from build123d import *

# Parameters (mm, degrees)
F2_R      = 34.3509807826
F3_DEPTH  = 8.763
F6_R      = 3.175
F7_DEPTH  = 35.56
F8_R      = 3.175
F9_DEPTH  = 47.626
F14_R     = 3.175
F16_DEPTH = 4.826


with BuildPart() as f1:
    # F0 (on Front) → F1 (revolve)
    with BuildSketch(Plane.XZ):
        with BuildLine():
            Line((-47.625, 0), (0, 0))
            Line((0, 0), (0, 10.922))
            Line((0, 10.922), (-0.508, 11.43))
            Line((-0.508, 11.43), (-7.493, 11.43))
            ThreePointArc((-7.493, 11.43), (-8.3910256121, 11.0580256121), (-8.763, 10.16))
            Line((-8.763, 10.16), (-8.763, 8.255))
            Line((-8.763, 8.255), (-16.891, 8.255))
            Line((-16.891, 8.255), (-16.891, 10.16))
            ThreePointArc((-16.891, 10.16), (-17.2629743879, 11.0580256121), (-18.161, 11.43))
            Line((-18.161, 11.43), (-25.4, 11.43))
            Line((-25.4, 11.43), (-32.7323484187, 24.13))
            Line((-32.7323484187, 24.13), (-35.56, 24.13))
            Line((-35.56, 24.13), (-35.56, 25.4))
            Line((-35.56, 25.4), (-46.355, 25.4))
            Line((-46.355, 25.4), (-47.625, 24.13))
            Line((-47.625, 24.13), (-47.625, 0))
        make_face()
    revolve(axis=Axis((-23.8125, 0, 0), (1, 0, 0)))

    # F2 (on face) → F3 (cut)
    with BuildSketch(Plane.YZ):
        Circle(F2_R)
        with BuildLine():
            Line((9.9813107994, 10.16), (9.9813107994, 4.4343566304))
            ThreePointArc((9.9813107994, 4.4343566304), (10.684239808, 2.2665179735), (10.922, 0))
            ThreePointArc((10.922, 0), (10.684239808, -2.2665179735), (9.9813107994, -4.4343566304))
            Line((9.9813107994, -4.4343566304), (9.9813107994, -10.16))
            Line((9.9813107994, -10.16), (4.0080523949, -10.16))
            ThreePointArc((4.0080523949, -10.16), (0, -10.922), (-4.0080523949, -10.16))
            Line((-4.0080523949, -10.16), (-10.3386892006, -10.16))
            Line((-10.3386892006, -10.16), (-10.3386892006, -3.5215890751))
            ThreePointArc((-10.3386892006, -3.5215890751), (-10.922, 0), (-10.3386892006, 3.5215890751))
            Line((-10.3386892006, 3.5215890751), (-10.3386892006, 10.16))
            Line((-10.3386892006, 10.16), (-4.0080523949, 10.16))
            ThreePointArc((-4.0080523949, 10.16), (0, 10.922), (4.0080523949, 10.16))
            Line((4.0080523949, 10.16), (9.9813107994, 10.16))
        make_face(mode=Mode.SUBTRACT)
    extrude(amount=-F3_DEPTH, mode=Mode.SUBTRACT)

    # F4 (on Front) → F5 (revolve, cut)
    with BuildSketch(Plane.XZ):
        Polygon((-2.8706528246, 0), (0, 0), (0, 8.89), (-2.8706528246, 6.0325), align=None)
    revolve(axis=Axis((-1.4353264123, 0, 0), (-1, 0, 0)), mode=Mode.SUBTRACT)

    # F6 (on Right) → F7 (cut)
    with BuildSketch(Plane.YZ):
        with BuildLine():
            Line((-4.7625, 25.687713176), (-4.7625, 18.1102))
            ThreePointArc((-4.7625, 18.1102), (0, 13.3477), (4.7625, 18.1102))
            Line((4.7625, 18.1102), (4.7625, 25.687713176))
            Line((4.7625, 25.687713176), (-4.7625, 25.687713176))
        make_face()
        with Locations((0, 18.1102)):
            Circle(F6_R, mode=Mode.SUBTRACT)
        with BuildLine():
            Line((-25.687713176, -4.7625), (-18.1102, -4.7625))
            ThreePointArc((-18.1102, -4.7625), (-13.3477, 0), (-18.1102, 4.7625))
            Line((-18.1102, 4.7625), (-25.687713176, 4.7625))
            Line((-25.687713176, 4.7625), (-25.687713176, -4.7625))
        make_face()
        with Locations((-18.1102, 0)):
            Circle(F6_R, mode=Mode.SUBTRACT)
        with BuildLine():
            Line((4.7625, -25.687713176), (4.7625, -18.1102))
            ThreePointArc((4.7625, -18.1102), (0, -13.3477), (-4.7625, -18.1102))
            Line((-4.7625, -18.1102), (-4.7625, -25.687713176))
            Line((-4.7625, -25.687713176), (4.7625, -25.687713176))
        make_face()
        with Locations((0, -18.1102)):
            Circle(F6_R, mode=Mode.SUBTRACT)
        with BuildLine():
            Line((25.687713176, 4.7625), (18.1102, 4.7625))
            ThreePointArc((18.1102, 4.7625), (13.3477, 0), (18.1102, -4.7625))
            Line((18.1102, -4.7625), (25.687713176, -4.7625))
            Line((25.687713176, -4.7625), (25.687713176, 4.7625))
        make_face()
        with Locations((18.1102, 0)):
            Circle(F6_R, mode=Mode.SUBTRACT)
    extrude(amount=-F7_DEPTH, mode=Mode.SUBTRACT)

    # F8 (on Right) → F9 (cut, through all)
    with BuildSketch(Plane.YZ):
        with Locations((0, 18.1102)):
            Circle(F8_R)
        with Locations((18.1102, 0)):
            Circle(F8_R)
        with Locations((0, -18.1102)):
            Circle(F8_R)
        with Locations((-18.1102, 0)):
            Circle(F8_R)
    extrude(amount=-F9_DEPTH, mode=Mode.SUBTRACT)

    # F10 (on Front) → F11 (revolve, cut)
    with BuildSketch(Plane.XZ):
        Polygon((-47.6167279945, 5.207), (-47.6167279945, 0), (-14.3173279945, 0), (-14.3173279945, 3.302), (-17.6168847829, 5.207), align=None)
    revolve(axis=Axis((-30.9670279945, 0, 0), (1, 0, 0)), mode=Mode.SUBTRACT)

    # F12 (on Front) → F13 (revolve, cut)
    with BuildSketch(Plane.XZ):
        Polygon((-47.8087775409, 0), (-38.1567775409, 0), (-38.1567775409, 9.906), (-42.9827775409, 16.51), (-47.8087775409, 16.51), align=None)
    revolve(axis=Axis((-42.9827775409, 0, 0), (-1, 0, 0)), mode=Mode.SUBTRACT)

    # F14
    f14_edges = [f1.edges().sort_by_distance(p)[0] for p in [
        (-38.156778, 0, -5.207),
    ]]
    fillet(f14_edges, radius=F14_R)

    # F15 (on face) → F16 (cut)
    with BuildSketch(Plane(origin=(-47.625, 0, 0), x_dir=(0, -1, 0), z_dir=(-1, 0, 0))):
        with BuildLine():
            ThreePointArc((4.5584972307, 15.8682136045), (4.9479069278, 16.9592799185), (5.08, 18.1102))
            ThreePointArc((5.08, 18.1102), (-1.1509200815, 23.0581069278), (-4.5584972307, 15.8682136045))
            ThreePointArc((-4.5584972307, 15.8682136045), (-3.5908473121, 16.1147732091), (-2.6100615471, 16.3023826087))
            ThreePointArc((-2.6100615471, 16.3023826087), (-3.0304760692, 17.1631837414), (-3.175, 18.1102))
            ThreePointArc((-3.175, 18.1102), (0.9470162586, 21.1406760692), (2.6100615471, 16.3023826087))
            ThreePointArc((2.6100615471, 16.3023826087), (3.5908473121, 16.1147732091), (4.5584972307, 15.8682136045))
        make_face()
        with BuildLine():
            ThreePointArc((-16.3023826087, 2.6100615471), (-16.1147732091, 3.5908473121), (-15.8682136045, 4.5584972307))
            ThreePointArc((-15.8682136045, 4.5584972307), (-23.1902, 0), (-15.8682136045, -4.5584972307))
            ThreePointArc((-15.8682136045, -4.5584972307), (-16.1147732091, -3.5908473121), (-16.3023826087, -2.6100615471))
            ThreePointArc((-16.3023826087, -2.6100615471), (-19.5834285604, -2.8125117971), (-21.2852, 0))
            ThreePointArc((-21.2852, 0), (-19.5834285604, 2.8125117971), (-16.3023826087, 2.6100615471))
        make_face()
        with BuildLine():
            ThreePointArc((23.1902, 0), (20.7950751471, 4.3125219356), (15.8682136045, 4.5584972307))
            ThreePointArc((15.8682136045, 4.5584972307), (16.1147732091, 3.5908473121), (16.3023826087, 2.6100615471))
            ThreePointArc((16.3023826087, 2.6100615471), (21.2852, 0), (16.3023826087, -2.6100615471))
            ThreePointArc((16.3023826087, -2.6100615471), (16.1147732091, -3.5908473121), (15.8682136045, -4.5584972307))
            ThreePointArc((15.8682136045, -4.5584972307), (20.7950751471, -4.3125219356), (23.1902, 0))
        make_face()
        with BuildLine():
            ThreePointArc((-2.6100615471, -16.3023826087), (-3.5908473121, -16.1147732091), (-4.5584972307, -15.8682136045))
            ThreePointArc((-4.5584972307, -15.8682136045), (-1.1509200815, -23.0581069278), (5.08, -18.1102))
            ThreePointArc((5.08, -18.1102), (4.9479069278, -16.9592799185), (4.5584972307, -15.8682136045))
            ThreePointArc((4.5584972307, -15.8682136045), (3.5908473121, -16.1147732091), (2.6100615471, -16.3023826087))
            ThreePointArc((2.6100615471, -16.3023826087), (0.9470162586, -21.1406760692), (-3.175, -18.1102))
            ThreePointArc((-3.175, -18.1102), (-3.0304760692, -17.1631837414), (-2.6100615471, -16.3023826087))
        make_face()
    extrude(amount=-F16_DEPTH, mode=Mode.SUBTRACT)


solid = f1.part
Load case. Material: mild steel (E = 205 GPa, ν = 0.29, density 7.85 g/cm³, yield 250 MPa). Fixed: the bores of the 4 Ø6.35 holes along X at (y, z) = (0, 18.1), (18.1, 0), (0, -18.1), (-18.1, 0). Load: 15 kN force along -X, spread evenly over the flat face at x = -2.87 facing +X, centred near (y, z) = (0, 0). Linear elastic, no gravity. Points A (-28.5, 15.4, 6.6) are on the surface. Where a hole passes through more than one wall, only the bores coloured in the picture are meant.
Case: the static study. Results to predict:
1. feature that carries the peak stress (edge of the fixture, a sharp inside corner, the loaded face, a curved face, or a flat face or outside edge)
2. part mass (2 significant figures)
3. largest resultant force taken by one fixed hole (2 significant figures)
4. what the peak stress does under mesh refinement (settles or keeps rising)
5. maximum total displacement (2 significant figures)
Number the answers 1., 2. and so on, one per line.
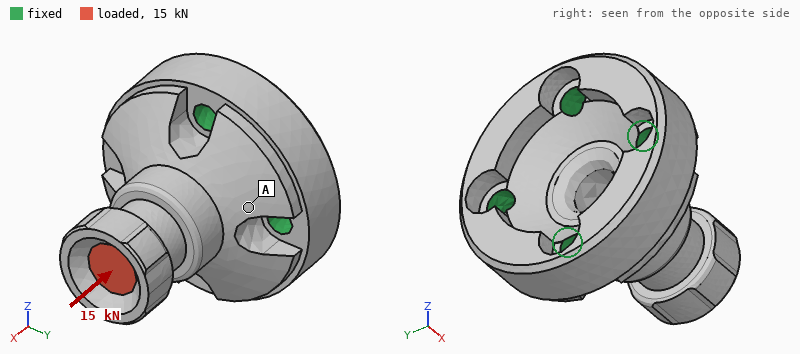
1. edge of the fixture
2. 250 g
3. 4.2 kN
4. keeps rising
5. 13 µm
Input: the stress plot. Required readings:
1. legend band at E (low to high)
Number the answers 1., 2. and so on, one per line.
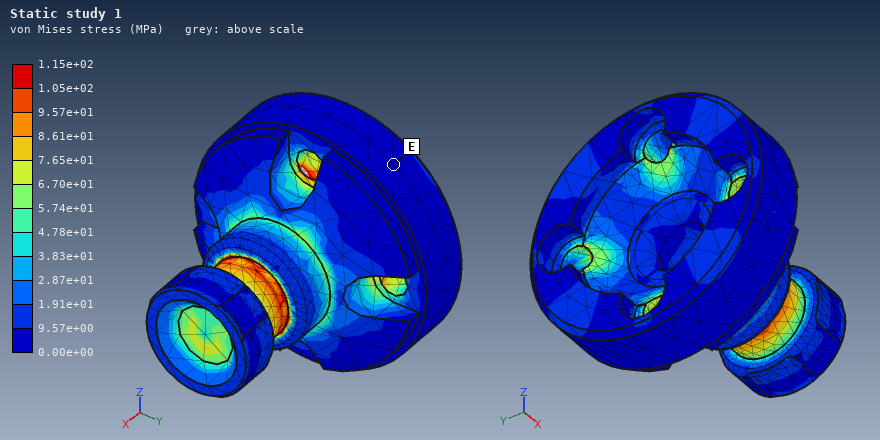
1. 0.00e+00 to 9.57e+00 MPa
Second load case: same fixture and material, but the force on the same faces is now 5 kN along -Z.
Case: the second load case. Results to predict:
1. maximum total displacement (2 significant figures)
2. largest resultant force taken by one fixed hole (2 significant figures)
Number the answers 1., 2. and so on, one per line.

1. 39 µm
2. 5.1 kN
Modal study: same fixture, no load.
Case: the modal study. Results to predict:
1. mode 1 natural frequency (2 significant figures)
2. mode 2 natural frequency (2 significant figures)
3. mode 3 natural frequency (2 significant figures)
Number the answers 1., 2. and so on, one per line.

1. 12 kHz
2. 12 kHz
3. 23 kHz
